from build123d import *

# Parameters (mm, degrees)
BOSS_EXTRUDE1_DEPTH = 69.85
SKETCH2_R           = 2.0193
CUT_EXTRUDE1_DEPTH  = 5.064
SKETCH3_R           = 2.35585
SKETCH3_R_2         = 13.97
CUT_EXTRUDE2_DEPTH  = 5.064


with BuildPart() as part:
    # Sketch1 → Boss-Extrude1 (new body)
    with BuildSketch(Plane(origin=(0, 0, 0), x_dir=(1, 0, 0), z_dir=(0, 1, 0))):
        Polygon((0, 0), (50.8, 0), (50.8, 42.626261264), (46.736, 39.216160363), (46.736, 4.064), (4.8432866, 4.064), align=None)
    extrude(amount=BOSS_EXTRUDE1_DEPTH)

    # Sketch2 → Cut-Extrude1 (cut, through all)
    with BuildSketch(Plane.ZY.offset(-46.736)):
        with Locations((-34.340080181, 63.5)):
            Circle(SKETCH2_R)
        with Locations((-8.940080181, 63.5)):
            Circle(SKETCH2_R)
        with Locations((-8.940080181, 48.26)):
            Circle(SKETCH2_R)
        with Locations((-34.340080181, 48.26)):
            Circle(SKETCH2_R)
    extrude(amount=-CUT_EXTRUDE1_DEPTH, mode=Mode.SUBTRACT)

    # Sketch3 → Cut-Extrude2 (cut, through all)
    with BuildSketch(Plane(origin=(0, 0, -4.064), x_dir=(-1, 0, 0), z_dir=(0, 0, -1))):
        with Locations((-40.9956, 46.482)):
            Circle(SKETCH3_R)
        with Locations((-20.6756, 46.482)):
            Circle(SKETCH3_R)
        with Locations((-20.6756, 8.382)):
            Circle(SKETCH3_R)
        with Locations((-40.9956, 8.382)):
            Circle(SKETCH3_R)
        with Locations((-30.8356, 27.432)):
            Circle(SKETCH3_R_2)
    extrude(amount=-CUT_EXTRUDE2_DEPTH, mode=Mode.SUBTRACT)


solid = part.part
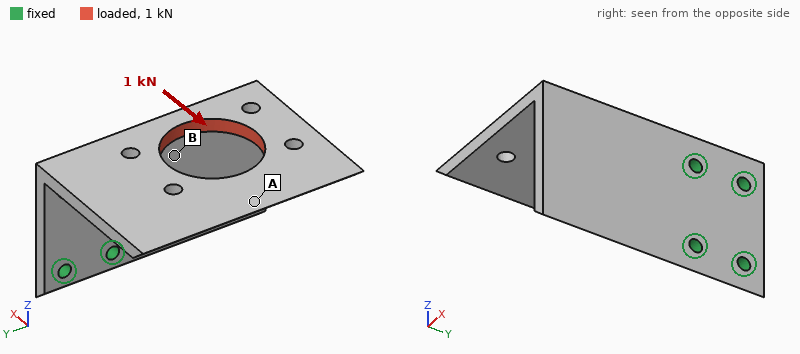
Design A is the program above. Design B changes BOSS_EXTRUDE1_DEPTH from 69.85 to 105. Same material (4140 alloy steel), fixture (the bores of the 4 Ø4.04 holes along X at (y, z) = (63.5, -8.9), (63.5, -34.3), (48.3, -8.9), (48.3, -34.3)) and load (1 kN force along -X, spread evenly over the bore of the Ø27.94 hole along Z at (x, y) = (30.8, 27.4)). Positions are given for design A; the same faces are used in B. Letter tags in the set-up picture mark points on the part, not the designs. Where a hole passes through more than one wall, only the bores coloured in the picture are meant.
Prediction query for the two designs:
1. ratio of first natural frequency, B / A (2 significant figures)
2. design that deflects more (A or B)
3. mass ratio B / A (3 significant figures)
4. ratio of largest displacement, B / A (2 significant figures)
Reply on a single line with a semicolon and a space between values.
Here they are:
1.0; A; 1.57; 0.80
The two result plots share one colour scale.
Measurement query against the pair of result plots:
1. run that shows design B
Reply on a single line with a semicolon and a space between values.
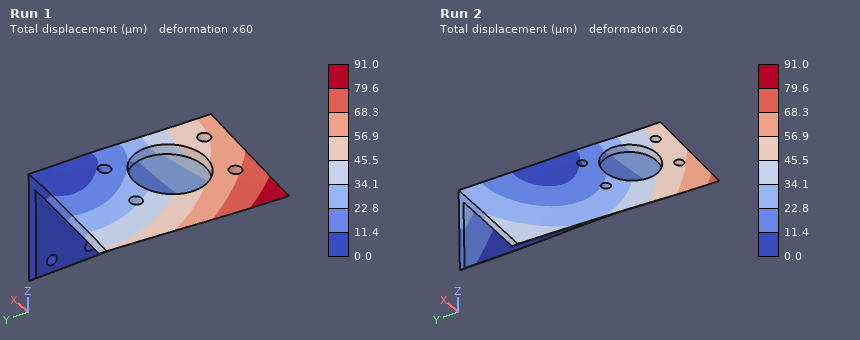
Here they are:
Run 2
